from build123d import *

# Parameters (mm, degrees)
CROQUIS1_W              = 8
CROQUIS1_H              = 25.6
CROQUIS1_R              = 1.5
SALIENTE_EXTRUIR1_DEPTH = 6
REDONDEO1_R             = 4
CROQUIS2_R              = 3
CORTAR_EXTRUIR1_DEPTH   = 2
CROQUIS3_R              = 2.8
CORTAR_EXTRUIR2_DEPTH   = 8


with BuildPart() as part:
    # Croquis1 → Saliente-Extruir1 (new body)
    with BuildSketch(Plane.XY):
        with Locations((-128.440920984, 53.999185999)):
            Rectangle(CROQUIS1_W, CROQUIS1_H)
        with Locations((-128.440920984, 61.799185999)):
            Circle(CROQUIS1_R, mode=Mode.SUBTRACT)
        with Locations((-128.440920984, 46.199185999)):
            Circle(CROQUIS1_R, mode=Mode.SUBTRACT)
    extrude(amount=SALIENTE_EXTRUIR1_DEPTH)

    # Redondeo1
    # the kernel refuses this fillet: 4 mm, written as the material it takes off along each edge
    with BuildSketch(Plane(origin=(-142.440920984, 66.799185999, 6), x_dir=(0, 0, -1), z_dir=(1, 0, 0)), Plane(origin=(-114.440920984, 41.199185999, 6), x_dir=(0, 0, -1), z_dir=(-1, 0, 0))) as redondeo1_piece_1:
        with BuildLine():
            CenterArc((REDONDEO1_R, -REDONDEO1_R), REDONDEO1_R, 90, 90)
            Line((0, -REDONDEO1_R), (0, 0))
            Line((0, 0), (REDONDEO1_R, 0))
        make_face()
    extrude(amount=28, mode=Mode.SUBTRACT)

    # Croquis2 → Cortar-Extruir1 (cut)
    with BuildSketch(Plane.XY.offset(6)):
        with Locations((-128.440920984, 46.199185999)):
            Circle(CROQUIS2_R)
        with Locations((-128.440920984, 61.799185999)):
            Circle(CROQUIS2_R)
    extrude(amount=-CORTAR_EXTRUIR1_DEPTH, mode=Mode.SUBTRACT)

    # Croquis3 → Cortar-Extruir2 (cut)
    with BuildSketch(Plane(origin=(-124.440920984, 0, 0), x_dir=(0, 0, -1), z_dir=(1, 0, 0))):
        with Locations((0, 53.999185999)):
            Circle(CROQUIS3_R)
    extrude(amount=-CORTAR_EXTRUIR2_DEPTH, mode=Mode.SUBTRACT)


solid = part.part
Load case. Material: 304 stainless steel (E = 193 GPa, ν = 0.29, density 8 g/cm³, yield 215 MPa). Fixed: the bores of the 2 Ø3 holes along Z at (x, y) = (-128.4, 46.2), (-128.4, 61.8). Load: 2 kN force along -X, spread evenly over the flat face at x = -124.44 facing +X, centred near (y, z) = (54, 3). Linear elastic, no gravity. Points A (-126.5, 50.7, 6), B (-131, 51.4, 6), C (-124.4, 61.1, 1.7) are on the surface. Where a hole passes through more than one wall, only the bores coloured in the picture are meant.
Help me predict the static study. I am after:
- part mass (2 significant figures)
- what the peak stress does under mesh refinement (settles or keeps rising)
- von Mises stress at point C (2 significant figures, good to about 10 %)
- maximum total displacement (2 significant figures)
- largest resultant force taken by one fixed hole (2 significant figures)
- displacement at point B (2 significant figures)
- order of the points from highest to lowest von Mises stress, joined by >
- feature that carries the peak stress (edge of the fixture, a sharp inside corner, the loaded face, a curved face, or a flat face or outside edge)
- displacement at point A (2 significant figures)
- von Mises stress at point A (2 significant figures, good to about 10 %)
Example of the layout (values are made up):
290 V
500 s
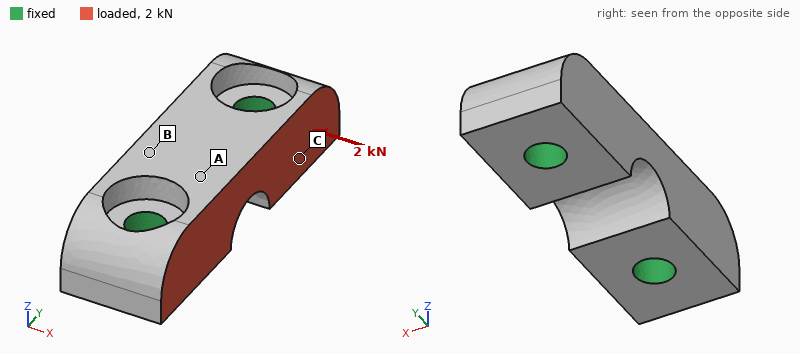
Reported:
7.3 g
keeps rising
38 MPa
2.6 µm
1.0 kN
1.9 µm
C > A > B
edge of the fixture
2.0 µm
21 MPa
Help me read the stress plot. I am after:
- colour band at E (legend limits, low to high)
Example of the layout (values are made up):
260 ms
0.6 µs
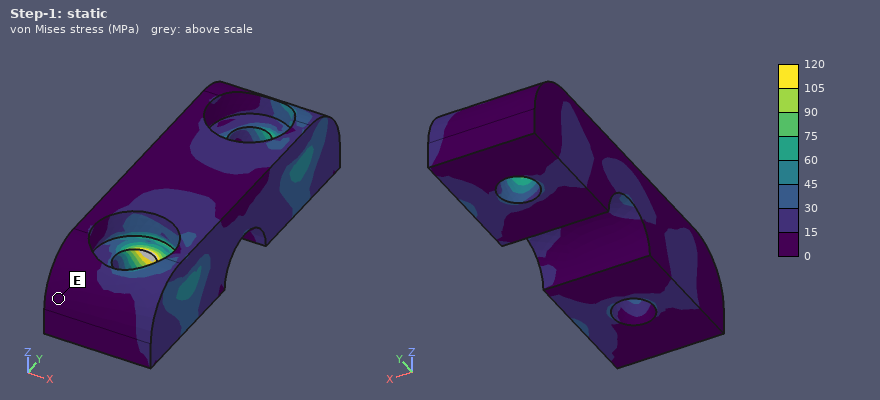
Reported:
0 to 15 MPa
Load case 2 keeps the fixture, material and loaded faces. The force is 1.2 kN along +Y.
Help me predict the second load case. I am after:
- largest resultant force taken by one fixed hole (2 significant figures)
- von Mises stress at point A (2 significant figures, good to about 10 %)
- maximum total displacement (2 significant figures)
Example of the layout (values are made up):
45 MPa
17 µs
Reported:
630 N
14 MPa
1.5 µm
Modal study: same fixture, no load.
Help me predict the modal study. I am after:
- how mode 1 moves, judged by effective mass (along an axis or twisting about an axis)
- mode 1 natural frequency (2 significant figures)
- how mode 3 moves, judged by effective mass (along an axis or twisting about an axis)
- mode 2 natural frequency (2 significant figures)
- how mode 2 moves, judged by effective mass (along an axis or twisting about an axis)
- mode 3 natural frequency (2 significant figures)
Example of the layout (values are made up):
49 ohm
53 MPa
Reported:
along X
59 kHz
twisting about Y
73 kHz
along Z
90 kHz
